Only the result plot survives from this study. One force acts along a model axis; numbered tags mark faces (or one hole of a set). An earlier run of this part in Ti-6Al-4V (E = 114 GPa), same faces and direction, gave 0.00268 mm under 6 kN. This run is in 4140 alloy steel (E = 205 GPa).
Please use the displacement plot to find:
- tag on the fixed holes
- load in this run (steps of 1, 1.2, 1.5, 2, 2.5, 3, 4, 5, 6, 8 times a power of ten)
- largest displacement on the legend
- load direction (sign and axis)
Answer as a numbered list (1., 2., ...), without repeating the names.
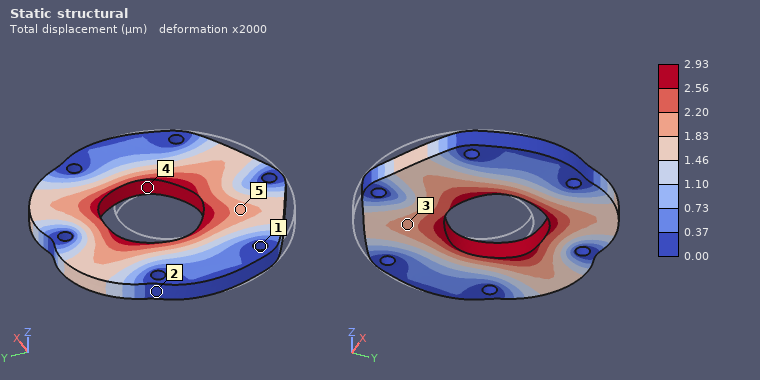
1. 1
2. 12 kN
3. 2.93 µm
4. +Y
